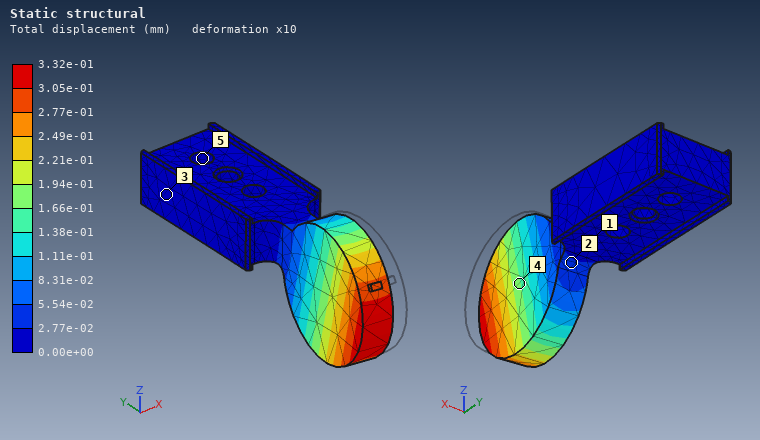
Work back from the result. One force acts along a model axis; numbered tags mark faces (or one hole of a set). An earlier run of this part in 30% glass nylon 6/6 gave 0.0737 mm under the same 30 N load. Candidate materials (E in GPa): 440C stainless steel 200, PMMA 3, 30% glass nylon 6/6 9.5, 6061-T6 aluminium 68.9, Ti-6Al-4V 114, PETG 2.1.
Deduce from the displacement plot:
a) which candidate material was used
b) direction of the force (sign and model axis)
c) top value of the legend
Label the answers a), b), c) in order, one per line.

a) PETG
b) -X
c) 3.32e-01 mm
